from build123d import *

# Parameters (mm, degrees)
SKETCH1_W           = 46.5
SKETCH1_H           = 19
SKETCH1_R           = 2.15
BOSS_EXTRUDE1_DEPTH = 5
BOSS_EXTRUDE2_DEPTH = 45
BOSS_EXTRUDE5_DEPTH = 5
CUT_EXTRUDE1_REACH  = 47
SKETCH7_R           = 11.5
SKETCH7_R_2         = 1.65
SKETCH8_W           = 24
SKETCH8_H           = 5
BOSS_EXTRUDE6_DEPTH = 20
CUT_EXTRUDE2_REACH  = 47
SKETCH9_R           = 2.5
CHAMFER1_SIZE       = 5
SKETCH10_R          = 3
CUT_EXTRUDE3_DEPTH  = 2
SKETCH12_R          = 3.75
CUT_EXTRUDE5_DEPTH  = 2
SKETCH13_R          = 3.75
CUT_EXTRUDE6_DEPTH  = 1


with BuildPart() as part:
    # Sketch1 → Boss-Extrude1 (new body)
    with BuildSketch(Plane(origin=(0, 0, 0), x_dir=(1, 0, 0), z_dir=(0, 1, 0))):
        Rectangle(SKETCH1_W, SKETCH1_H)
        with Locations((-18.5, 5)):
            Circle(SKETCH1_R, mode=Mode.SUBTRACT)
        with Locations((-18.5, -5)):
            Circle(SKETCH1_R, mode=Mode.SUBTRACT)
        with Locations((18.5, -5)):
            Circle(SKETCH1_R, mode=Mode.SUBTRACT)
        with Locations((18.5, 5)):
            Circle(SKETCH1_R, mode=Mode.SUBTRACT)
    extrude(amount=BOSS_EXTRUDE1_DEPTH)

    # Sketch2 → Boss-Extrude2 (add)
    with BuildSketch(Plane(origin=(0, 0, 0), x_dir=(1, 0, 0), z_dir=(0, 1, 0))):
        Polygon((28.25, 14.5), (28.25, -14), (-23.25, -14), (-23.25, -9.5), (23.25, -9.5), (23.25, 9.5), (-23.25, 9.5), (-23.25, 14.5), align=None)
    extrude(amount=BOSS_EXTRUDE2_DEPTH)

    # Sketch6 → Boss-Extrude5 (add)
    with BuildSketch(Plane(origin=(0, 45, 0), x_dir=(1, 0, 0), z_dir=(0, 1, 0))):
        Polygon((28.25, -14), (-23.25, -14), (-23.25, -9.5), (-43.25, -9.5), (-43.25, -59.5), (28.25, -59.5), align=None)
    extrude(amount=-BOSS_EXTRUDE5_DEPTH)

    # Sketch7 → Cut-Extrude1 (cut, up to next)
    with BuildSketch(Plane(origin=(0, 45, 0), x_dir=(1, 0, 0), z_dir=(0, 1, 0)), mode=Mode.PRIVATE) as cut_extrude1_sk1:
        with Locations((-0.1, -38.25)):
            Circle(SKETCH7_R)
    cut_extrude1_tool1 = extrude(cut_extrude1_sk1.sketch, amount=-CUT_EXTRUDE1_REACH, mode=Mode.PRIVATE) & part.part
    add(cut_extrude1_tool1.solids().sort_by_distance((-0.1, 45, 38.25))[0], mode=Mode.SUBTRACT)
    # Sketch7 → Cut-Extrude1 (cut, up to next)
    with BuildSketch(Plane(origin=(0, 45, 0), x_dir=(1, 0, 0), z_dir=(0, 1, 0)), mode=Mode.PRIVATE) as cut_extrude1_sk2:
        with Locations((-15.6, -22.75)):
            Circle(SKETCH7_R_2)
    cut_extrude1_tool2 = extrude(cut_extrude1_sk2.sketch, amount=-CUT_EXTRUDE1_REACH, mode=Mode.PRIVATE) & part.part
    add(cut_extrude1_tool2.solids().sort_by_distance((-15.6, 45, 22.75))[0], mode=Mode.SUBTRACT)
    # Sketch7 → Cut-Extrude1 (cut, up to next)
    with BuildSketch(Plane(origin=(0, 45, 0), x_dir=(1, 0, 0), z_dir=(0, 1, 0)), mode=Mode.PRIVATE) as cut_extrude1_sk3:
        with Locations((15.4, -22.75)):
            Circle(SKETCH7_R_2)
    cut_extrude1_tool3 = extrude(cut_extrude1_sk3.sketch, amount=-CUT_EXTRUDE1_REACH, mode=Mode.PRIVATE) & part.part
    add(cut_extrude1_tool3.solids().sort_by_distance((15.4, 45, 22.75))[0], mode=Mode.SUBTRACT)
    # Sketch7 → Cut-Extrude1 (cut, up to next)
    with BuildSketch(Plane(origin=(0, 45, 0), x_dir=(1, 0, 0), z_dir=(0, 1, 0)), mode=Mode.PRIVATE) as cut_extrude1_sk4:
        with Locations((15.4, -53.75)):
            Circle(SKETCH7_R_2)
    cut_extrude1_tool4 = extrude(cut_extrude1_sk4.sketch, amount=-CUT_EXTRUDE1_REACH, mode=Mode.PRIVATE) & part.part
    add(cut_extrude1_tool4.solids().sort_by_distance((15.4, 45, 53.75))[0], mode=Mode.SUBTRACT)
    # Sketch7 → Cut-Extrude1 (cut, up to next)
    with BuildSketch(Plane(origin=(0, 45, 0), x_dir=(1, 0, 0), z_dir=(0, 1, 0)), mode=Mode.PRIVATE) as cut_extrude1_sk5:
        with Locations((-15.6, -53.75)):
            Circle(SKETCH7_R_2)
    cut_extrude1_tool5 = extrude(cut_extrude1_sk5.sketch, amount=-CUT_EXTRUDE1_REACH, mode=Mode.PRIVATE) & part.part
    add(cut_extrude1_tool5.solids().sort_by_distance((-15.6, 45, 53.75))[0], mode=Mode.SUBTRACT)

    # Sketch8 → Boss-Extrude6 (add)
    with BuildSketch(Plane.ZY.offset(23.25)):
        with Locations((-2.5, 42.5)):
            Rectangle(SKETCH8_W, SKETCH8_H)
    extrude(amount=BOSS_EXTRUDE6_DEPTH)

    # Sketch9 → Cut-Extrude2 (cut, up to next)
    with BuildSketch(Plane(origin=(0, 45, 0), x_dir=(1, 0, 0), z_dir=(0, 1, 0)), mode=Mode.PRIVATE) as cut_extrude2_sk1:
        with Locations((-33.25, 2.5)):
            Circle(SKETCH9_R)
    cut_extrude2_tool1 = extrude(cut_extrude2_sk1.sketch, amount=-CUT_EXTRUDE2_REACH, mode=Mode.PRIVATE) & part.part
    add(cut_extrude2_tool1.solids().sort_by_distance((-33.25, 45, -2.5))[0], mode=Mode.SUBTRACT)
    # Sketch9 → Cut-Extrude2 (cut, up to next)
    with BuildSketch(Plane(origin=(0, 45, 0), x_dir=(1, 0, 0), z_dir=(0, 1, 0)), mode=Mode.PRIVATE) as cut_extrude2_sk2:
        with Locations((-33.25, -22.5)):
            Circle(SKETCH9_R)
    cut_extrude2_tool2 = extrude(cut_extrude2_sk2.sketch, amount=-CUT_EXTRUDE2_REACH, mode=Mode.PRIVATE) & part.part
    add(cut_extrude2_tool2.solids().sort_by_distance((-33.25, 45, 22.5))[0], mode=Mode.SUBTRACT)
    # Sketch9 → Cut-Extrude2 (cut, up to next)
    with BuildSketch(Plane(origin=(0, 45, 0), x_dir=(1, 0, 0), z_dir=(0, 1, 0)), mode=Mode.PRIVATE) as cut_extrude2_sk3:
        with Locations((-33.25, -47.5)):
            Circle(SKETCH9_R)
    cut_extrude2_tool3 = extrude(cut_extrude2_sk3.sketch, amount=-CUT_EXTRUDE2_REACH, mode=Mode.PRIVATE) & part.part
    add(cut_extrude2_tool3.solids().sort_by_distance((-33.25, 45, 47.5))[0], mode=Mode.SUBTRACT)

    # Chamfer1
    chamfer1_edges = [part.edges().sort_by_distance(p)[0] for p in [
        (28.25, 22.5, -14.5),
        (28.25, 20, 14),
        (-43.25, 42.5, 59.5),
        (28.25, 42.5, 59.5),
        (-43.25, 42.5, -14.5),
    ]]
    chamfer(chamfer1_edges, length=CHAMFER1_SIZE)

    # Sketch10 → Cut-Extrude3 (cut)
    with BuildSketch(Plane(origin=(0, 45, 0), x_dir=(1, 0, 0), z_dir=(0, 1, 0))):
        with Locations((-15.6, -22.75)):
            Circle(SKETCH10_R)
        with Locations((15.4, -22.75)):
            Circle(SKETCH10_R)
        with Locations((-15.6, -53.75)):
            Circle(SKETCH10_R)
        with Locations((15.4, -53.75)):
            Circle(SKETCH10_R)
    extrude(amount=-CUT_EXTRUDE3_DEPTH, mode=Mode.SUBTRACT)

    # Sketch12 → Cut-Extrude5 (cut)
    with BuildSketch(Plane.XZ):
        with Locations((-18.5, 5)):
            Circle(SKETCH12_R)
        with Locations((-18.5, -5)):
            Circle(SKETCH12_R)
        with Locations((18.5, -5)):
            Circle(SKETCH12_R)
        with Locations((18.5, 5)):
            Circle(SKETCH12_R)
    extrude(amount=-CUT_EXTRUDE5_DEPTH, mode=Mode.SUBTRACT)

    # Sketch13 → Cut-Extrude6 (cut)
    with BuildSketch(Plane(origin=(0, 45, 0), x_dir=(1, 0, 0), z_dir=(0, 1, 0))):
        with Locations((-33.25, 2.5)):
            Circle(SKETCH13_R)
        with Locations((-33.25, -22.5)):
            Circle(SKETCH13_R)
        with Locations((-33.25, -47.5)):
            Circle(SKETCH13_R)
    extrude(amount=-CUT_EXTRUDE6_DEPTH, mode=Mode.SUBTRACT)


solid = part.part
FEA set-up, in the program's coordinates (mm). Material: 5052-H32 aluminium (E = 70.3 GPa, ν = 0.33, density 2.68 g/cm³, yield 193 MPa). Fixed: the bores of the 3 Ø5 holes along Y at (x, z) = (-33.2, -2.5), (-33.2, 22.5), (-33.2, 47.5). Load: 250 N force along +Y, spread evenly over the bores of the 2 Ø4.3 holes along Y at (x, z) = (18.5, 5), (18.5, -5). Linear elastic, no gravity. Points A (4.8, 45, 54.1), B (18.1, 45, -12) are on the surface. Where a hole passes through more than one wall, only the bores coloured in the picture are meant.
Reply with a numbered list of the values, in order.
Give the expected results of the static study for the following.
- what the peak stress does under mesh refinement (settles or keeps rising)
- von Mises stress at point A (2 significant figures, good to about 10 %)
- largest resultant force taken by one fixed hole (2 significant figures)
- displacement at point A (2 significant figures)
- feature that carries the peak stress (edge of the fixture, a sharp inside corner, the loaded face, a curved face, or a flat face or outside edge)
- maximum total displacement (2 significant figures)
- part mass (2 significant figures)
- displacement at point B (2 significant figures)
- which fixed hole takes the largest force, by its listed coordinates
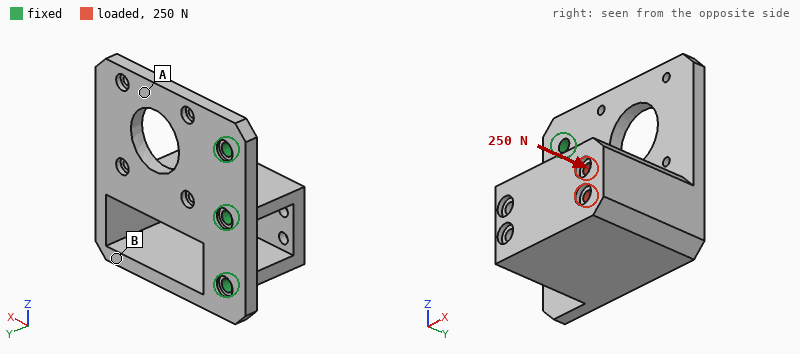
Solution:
1. keeps rising
2. 17 MPa
3. 180 N
4. 0.10 mm
5. edge of the fixture
6. 0.43 mm
7. 120 g
8. 0.29 mm
9. (-33.2, -2.5)
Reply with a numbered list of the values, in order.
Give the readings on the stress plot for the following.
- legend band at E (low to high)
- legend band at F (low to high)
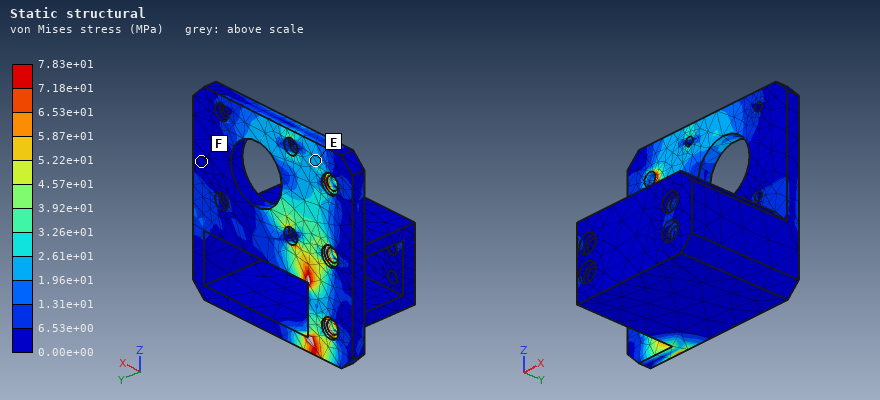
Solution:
1. 1.96e+01 to 2.61e+01 MPa
2. 0.00e+00 to 6.53e+00 MPa
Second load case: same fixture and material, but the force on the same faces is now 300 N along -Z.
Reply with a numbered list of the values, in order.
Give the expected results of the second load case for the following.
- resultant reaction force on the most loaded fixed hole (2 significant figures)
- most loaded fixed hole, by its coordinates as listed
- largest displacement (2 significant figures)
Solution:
1. 470 N
2. (-33.2, -2.5)
3. 0.14 mm
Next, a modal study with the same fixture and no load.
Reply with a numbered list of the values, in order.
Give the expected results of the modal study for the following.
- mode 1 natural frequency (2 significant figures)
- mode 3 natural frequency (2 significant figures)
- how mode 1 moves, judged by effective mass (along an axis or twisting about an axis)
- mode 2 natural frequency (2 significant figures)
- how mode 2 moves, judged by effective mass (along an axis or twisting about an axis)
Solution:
1. 530 Hz
2. 2700 Hz
3. along Y
4. 1300 Hz
5. along Z
